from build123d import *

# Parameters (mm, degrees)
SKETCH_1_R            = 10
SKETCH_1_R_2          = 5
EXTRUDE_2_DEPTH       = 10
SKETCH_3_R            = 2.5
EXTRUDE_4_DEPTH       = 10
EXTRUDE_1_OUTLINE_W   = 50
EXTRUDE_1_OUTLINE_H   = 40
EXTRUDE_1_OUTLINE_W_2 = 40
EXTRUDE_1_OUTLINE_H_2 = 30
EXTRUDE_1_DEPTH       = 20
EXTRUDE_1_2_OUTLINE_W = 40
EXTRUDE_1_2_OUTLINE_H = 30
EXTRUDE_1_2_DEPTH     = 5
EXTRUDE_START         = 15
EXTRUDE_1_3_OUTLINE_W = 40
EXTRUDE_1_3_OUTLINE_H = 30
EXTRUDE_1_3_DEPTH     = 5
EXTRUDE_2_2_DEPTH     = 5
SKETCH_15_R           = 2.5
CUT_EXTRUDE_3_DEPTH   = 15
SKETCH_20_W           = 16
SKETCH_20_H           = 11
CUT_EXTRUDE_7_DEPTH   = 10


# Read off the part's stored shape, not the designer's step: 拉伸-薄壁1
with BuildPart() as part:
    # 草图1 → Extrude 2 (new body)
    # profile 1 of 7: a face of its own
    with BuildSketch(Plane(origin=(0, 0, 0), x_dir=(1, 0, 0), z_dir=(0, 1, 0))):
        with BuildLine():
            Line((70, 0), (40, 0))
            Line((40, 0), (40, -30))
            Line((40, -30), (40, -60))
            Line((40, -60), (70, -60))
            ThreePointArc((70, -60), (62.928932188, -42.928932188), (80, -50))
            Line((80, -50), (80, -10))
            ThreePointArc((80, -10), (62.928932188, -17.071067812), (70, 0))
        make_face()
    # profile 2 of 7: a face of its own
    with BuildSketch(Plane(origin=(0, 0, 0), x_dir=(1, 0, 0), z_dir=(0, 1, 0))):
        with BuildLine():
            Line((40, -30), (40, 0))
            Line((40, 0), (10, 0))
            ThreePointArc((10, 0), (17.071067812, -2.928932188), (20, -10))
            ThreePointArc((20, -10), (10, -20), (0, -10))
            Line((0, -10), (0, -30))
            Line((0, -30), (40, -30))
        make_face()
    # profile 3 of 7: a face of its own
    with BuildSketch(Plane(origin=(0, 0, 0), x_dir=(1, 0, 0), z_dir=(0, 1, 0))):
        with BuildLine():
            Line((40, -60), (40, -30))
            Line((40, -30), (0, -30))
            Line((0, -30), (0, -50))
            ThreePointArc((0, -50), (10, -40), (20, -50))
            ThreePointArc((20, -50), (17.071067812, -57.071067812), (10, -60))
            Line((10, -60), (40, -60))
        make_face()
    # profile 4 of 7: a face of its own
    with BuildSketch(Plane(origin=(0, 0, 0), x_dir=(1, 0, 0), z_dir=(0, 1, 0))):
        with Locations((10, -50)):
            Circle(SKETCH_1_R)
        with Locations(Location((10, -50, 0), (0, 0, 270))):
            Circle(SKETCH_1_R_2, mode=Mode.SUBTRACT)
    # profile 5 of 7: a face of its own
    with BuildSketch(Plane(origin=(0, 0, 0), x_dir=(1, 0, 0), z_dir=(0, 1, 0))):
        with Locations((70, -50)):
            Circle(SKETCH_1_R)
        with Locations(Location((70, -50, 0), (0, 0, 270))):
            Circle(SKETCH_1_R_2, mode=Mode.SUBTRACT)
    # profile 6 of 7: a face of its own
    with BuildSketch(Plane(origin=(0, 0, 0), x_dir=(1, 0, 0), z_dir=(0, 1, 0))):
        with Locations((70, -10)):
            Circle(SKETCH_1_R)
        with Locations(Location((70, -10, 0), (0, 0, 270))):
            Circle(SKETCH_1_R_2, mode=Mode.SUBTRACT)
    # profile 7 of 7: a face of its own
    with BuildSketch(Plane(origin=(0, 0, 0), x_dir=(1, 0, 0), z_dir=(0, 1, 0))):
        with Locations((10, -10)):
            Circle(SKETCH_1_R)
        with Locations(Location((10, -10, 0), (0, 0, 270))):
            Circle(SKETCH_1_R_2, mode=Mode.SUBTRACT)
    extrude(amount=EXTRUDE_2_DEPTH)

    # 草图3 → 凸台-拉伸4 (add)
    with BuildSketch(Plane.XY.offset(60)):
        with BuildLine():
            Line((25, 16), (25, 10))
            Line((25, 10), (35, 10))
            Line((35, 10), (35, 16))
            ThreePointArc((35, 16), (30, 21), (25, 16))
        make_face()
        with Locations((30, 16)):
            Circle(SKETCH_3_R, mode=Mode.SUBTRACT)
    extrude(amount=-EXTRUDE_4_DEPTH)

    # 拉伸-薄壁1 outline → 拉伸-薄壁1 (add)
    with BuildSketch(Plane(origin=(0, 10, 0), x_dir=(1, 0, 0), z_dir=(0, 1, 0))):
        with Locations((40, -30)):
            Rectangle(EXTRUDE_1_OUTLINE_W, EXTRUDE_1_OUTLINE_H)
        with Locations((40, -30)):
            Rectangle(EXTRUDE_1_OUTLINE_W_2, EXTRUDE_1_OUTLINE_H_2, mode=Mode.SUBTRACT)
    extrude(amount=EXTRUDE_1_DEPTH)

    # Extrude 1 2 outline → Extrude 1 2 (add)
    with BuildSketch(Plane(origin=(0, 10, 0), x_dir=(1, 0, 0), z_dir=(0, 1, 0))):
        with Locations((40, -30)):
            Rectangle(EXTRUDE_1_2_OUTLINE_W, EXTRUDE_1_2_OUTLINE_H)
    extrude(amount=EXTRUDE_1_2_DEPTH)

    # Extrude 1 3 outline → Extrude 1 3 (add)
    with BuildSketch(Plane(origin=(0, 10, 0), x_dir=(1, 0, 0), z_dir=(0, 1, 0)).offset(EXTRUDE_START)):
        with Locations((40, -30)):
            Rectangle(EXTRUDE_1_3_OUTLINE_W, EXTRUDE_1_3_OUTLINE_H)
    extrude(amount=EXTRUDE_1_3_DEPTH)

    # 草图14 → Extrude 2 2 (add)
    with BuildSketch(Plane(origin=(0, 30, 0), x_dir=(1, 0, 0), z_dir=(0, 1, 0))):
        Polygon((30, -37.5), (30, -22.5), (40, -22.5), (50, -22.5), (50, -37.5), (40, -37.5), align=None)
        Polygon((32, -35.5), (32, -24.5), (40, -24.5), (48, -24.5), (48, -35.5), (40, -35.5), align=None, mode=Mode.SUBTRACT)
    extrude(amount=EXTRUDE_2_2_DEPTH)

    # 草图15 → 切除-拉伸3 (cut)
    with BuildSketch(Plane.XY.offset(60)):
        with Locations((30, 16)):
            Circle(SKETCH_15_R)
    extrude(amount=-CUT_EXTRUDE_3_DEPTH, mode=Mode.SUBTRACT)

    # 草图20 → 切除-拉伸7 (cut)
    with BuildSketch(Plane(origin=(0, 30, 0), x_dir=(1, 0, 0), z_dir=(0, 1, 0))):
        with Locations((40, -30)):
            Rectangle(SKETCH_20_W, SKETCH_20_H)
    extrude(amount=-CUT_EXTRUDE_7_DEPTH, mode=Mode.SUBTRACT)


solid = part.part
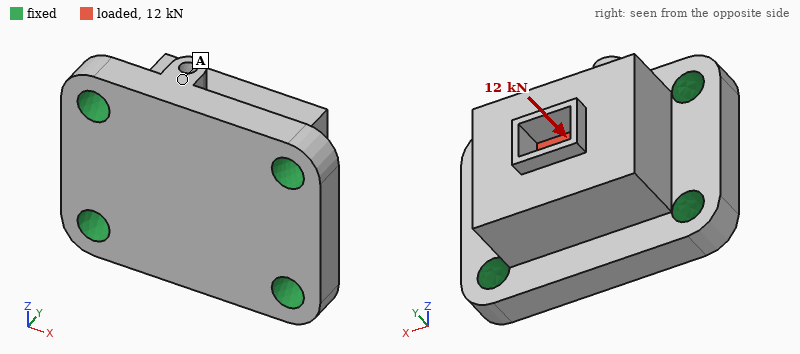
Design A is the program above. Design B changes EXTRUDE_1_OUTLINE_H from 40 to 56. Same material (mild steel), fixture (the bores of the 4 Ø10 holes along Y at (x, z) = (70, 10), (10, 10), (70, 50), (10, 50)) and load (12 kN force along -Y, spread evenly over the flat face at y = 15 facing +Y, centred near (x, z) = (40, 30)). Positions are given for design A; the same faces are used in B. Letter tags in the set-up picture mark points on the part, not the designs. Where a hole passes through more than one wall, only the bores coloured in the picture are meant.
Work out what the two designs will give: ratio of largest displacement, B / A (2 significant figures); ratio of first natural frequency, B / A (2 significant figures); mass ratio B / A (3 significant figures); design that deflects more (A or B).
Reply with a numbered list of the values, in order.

1. 0.83
2. 0.96
3. 1.21
4. A
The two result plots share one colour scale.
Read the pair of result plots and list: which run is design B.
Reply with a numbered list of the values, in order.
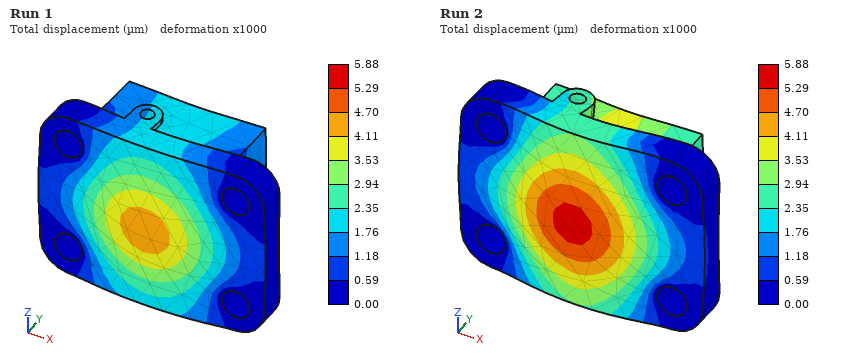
1. Run 1
